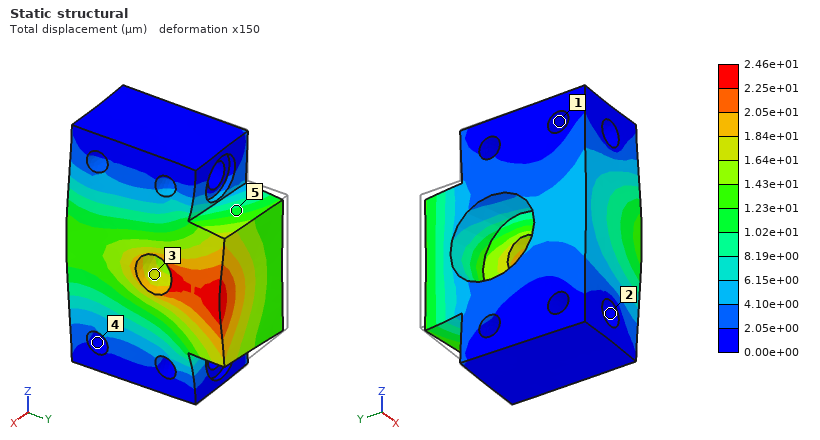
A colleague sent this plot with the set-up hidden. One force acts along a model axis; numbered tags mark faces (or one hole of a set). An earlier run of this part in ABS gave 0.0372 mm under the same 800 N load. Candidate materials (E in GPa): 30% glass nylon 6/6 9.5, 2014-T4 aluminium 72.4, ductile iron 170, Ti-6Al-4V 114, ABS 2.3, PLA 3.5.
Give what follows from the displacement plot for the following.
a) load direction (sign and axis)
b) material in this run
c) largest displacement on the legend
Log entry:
-Y
PLA
2.46e+01 µm
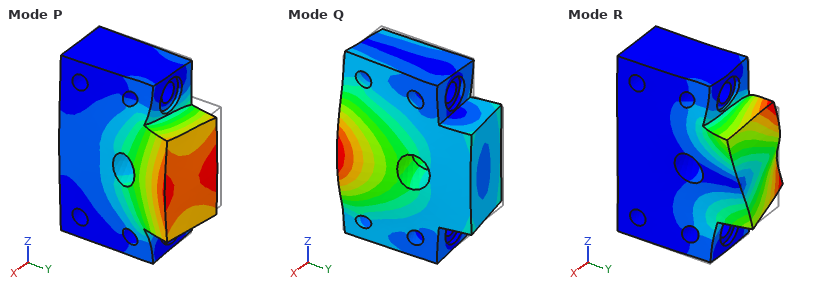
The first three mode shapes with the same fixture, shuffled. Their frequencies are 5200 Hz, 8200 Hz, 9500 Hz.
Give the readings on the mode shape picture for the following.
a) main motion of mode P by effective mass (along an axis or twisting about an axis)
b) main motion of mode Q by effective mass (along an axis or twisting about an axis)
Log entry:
along X
along X
